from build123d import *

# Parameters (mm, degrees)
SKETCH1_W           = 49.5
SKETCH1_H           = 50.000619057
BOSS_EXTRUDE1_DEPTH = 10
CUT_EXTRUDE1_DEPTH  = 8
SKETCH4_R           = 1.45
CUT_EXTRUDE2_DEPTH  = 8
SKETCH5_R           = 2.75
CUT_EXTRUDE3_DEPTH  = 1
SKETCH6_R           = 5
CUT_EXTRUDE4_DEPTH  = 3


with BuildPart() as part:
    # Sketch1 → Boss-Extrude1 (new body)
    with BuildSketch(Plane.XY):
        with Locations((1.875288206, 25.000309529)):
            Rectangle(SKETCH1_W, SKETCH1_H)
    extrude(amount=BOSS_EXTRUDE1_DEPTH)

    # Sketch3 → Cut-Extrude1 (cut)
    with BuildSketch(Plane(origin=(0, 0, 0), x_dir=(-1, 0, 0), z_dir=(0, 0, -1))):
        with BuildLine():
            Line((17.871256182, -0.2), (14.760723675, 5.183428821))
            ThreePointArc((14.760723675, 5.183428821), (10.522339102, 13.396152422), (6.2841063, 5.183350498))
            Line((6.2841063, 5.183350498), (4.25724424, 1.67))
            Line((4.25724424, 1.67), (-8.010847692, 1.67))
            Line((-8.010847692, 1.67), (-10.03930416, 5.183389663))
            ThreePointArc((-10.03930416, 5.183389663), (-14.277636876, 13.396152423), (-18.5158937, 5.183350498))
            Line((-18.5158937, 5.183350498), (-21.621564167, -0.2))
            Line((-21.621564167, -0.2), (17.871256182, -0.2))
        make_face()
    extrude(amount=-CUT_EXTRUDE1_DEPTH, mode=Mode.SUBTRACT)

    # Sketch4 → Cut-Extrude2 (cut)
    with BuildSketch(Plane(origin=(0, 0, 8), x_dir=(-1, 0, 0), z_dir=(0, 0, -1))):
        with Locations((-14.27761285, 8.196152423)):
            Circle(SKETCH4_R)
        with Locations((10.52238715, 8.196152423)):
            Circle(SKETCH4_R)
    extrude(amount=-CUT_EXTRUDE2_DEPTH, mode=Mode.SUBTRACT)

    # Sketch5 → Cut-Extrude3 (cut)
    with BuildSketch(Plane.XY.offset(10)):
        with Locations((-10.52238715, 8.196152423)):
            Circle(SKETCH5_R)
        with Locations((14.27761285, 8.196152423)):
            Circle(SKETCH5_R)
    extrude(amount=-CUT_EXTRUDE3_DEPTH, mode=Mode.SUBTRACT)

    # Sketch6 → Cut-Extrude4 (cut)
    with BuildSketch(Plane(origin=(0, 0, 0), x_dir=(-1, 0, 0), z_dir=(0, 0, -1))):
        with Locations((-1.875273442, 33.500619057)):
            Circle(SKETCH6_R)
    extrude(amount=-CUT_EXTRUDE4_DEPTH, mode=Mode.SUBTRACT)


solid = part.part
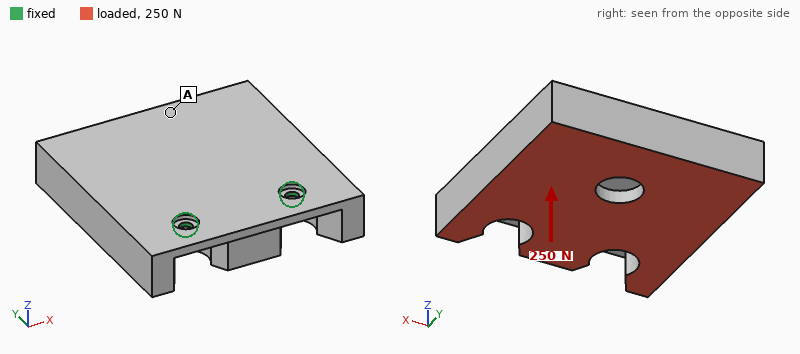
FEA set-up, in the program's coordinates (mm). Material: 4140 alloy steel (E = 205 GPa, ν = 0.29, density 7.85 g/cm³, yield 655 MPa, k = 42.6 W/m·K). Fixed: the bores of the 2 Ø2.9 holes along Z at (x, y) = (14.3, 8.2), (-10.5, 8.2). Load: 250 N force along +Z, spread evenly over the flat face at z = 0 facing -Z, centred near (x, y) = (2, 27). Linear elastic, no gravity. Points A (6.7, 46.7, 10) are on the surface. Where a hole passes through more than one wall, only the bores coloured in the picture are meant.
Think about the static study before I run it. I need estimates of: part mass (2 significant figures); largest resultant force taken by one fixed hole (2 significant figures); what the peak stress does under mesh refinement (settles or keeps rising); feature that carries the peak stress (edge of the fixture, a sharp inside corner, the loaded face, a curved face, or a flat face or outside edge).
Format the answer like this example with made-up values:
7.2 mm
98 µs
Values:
170 g
130 N
keeps rising
edge of the fixture
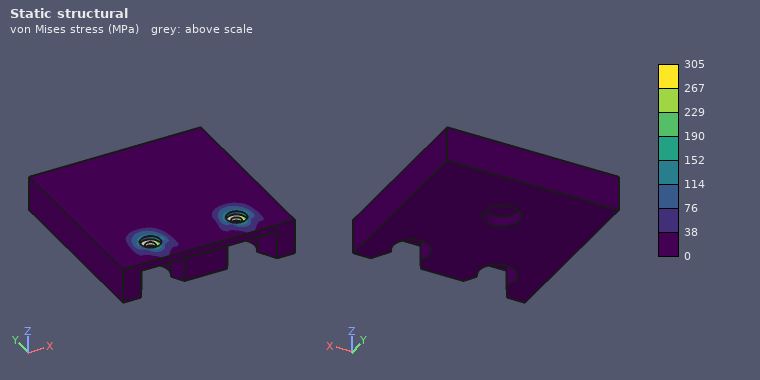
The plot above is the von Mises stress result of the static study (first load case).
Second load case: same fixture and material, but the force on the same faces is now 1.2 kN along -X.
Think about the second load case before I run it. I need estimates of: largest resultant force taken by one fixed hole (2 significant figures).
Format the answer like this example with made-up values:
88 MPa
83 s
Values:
1.1 kN
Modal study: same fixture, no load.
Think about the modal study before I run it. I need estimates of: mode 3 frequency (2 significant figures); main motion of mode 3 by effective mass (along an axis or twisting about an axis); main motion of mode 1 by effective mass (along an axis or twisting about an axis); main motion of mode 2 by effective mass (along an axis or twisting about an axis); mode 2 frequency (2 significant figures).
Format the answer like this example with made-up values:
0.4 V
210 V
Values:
4700 Hz
along X
along Z
twisting about Y
3900 Hz
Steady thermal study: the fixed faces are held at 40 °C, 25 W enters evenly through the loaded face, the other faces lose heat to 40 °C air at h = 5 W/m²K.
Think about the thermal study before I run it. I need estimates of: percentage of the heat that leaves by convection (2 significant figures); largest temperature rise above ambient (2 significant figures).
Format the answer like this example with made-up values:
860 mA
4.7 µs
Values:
6.5 %
77 K
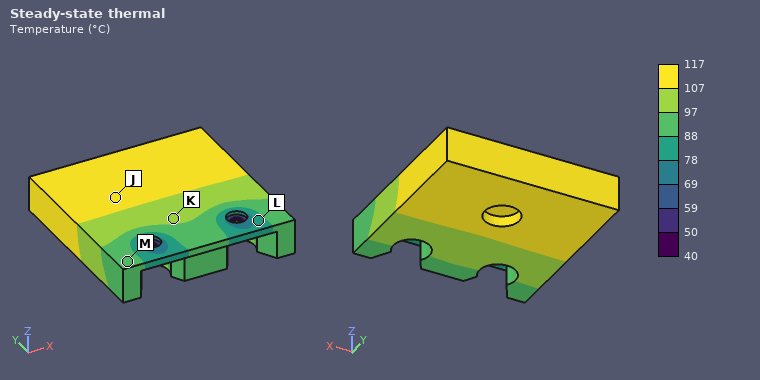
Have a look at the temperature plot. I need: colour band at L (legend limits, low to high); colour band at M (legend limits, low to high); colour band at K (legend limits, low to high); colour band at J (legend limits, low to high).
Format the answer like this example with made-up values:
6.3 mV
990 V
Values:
78 to 88 °C
88 to 97 °C
97 to 107 °C
107 to 117 °C
